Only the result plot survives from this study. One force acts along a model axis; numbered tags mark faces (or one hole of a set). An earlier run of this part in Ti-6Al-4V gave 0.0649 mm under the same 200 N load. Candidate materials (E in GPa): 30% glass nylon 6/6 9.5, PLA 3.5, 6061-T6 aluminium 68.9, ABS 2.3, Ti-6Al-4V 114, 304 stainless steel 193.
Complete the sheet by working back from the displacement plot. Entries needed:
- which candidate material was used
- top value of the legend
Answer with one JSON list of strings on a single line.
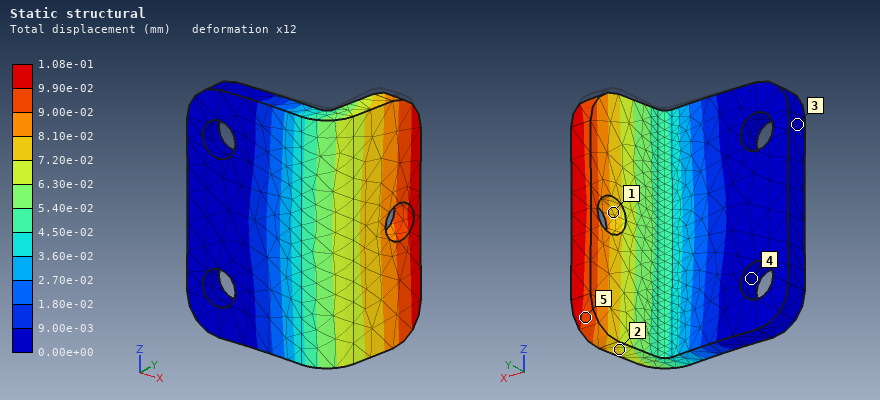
["6061-T6 aluminium", "1.08e-01 mm"]
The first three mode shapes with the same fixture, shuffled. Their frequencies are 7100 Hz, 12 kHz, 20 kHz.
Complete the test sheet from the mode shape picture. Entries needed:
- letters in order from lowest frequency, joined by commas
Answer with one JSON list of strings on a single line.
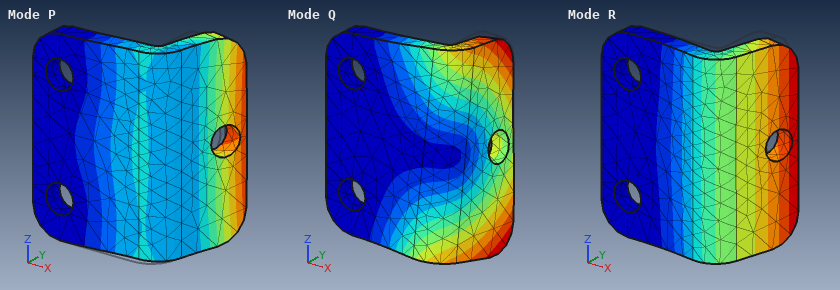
["R, Q, P"]
